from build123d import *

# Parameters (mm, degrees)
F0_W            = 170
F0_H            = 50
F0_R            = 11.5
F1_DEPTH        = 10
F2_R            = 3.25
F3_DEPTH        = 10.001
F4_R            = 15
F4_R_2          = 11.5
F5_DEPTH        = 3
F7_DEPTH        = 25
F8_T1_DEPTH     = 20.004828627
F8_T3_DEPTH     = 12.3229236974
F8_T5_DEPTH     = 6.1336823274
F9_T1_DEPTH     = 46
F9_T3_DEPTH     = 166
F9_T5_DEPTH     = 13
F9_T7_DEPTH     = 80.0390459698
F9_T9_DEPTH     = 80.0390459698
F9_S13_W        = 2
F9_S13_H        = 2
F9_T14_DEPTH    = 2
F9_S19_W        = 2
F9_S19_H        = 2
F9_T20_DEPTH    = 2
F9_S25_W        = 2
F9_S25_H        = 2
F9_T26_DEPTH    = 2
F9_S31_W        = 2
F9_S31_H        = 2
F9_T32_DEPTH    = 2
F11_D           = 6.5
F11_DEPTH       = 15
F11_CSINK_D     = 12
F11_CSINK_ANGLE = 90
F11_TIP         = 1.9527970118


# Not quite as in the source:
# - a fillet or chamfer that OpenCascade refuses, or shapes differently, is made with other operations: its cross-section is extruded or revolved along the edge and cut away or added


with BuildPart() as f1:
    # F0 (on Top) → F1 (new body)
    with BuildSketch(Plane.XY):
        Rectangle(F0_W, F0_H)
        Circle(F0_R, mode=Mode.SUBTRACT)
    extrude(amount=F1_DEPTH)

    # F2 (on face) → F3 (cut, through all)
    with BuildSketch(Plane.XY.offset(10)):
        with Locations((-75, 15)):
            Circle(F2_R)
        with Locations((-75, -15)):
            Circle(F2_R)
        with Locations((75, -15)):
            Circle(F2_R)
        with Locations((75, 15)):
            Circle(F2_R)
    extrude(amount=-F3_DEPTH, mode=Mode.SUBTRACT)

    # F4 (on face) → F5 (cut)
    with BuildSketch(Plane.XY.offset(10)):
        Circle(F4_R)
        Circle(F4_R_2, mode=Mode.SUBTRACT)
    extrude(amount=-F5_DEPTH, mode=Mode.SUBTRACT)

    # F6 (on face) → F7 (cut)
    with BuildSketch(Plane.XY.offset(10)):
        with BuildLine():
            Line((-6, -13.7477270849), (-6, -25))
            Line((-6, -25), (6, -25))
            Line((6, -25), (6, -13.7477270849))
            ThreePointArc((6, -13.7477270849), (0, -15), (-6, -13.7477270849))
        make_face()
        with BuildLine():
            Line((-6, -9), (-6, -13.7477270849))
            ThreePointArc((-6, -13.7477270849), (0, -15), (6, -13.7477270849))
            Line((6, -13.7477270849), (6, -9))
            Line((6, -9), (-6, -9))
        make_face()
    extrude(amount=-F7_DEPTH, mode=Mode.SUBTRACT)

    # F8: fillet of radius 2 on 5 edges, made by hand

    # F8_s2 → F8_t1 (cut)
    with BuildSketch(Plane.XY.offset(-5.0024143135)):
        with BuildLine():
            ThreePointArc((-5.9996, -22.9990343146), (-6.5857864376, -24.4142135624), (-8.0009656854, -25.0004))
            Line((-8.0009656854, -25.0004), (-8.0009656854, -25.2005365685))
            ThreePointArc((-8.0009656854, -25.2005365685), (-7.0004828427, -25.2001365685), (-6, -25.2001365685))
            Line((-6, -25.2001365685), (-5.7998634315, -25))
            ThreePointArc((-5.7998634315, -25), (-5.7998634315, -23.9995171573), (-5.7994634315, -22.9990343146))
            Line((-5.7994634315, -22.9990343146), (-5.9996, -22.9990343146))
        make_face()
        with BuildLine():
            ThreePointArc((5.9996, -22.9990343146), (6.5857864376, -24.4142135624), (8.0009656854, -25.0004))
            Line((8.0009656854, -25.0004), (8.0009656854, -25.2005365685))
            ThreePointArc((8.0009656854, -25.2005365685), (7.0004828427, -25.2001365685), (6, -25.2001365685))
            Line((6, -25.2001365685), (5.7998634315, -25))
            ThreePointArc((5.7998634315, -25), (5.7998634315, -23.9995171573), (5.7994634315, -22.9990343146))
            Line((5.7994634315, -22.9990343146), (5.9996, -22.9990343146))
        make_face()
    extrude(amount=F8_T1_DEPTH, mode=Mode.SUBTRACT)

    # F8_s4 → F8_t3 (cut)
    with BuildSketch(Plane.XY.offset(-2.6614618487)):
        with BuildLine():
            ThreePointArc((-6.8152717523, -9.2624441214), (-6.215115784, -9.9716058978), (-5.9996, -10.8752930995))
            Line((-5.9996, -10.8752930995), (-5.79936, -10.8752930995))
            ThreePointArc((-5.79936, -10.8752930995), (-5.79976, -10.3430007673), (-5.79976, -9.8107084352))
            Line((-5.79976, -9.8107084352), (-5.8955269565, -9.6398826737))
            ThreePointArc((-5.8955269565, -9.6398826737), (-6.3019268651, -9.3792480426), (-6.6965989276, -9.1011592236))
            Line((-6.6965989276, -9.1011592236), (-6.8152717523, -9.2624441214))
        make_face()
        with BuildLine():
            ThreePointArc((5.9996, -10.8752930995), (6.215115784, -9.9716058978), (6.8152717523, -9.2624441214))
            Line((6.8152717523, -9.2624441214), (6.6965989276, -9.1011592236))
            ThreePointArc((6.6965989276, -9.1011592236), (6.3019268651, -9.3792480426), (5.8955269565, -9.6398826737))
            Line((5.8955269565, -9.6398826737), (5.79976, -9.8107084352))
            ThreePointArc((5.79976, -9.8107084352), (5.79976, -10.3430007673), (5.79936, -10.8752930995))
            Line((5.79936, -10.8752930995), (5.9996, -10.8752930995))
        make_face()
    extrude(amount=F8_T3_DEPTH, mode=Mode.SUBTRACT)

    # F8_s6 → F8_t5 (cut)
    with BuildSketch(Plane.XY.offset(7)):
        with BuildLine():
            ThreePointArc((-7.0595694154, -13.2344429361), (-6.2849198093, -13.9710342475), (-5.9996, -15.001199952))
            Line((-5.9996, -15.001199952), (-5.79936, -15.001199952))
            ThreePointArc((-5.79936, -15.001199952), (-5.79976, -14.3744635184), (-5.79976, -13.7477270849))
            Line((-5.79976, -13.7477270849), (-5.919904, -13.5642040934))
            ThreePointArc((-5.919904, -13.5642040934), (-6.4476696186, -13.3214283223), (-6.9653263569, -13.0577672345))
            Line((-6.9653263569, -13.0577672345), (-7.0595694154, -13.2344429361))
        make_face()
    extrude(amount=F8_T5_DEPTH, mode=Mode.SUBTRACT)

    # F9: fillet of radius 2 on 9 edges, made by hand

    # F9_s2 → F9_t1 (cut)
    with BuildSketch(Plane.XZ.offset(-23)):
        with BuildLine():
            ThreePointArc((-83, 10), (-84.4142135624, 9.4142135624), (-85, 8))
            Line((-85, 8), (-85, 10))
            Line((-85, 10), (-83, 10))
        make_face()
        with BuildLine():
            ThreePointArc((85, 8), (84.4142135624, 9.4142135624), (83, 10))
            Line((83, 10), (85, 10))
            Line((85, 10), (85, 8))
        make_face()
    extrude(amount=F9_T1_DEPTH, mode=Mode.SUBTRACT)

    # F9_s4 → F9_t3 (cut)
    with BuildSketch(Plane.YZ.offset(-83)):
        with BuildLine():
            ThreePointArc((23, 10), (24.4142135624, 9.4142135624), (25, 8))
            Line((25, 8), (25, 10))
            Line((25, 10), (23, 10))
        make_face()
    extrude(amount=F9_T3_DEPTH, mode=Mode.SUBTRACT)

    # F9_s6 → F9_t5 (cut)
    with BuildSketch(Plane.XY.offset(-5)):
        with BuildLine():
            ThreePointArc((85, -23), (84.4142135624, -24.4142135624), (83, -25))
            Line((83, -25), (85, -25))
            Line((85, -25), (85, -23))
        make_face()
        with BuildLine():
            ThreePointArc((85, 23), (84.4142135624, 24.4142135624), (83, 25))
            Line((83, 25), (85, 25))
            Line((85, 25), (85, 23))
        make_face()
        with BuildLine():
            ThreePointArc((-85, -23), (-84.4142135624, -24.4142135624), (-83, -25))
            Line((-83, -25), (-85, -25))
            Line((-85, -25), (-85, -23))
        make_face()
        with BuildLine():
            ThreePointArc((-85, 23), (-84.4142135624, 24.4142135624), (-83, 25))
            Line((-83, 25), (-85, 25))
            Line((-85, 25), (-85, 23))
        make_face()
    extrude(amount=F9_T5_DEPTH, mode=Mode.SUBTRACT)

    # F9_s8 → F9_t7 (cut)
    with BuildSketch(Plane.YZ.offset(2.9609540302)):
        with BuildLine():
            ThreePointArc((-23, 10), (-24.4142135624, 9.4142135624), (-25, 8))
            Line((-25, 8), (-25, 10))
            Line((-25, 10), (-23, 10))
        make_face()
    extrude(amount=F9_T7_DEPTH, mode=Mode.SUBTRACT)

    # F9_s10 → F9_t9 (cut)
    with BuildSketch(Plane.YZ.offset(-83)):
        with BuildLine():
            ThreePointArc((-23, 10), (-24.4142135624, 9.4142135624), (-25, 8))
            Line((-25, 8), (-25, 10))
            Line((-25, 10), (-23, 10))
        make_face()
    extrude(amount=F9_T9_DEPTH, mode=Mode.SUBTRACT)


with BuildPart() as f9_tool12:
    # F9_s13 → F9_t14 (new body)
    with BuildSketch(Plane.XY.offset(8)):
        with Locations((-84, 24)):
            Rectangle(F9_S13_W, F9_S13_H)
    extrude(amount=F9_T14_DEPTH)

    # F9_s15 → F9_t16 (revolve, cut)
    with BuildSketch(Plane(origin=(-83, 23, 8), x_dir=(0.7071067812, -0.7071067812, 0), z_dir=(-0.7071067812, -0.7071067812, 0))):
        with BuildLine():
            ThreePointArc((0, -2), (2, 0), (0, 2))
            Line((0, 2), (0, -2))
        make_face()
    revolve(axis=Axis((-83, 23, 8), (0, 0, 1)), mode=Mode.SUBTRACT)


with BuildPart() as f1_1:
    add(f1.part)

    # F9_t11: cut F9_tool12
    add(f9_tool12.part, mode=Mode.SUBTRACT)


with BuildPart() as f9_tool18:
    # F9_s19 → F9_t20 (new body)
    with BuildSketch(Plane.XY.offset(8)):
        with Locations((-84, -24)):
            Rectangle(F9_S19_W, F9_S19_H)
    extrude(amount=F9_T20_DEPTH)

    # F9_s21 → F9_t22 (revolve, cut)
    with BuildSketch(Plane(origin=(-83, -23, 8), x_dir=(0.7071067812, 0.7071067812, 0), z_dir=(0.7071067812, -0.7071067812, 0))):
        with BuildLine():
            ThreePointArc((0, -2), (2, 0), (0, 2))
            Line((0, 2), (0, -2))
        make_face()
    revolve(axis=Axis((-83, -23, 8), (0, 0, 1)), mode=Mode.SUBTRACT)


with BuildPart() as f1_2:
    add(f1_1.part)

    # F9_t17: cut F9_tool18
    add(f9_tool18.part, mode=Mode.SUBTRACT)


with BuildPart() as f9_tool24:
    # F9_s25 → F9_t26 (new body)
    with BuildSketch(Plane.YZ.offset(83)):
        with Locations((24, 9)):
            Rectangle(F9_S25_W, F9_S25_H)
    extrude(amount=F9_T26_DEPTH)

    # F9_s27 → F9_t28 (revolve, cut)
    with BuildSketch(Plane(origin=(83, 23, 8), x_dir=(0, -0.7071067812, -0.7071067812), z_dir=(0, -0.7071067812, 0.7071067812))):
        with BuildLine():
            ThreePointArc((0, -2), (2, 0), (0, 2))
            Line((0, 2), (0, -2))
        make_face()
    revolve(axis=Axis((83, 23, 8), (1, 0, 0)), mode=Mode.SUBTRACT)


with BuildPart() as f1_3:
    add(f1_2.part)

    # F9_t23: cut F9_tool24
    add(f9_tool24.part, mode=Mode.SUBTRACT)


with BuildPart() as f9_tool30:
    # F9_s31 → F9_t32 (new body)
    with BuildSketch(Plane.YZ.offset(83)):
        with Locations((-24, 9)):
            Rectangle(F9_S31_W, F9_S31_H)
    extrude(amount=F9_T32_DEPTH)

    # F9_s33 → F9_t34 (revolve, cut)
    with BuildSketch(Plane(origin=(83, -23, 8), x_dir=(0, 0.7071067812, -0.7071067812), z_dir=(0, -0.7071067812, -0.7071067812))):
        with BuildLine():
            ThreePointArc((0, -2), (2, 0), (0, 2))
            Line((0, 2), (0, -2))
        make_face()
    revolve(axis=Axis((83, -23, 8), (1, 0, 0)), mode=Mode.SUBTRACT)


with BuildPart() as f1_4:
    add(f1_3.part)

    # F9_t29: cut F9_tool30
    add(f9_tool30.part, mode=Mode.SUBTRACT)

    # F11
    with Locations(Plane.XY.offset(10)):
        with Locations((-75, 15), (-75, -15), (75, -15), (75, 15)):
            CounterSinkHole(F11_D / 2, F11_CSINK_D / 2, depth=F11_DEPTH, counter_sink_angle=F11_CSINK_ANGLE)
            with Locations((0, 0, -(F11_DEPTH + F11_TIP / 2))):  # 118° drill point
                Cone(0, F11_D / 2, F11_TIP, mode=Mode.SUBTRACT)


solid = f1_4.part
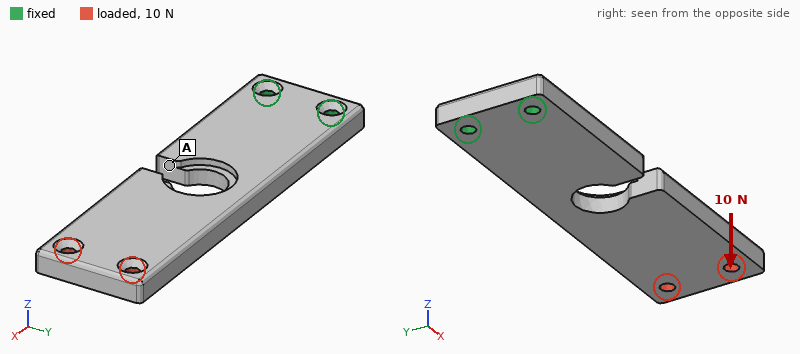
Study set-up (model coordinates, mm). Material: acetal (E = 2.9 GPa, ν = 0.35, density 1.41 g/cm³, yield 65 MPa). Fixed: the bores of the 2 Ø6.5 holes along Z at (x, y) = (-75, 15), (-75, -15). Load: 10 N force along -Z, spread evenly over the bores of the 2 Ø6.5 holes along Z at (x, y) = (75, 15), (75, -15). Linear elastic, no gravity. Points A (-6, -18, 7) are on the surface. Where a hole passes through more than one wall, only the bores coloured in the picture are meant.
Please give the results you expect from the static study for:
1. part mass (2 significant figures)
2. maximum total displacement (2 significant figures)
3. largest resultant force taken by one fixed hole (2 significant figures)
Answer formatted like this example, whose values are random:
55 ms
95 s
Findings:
110 g
1.9 mm
6.4 N
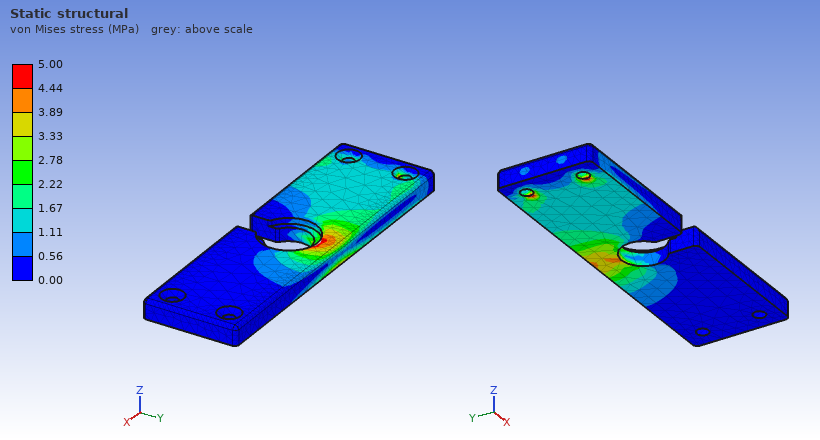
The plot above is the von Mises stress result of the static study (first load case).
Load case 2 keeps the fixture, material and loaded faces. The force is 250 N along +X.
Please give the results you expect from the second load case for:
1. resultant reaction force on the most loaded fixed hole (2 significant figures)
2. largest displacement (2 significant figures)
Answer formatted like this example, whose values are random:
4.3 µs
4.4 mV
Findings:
130 N
2.1 mm
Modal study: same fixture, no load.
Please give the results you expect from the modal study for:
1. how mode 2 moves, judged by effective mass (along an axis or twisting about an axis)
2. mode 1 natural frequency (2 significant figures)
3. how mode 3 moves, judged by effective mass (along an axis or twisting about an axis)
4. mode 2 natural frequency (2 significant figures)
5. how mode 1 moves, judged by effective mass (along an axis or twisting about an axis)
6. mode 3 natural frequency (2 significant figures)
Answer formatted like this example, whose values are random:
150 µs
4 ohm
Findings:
along Y
73 Hz
twisting about X
160 Hz
along Z
330 Hz
